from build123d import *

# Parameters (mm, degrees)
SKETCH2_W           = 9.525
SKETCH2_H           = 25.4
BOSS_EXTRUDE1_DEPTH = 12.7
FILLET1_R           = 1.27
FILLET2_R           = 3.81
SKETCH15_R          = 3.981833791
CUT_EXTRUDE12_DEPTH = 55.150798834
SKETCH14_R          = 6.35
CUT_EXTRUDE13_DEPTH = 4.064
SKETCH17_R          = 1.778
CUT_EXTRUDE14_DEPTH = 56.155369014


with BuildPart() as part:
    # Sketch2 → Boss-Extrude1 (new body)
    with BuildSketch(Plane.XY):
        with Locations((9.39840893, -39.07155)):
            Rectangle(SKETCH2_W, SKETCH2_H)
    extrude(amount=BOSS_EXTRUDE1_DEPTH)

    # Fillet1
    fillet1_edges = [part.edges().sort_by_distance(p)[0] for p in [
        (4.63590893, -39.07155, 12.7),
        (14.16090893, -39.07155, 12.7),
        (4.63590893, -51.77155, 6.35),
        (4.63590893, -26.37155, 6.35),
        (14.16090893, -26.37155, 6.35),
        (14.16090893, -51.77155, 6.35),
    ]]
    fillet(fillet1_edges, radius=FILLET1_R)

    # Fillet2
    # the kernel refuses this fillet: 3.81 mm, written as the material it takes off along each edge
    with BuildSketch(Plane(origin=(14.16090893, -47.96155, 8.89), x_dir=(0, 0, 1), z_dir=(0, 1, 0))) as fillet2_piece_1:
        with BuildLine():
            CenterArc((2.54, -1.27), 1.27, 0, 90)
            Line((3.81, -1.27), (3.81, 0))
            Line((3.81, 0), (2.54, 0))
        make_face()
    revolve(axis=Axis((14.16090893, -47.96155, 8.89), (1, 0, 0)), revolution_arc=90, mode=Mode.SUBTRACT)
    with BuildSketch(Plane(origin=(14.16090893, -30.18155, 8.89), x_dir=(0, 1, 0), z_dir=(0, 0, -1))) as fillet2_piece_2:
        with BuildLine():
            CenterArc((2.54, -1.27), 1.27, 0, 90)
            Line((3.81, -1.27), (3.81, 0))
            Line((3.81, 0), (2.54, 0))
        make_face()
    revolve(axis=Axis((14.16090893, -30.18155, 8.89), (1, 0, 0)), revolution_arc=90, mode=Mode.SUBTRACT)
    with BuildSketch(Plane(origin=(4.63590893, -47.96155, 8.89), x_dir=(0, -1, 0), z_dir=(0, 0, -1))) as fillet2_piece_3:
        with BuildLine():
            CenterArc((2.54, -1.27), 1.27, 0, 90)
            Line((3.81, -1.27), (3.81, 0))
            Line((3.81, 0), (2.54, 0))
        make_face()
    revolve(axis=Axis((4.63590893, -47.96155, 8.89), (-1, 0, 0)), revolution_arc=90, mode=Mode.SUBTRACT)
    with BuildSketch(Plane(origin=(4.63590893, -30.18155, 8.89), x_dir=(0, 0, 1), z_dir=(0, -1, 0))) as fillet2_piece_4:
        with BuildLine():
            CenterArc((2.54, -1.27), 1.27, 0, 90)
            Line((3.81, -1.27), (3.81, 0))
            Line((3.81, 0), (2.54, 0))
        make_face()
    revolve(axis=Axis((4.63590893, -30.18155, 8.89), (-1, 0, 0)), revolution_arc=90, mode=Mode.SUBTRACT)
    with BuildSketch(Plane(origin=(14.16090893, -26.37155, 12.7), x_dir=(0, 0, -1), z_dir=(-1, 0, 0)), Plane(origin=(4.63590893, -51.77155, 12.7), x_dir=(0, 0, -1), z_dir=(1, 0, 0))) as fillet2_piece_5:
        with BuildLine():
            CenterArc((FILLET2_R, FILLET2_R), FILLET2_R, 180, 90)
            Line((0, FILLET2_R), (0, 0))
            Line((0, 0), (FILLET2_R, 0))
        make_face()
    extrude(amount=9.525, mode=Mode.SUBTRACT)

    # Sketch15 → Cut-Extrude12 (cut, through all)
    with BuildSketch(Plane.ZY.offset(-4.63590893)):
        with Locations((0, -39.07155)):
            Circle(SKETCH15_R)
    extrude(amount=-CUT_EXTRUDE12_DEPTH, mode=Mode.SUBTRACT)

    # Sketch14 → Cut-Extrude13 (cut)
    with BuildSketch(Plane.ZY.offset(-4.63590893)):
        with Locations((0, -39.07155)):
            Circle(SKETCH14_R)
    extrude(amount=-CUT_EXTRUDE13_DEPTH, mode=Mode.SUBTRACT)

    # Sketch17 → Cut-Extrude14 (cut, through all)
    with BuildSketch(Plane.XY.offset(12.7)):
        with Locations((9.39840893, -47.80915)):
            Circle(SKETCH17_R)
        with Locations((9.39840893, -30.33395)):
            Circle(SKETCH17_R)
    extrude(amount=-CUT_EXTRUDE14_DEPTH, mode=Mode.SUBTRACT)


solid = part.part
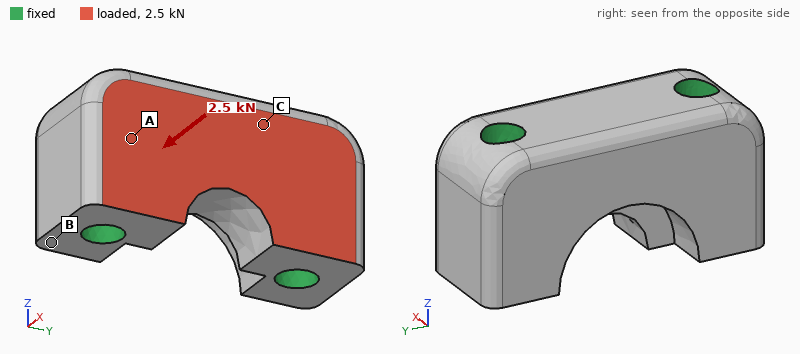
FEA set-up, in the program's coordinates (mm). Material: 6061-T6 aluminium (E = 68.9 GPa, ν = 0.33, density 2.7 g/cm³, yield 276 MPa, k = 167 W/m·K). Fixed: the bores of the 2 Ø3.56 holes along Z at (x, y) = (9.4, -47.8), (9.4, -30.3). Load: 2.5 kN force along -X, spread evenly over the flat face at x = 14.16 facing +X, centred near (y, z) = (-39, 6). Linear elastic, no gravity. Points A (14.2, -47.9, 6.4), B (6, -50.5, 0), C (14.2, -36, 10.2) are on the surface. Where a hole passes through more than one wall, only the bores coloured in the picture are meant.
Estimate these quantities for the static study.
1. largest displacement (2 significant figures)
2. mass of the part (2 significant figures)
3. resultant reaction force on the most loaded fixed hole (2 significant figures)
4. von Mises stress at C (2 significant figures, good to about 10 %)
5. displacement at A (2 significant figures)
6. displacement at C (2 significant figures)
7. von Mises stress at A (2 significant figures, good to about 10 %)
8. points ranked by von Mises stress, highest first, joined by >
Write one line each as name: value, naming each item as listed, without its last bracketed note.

largest displacement: 2.6 µm
mass of the part: 6.3 g
resultant reaction force on the most loaded fixed hole: 1.3 kN
von Mises stress at C: 7.5 MPa
displacement at A: 0.69 µm
displacement at C: 1.9 µm
von Mises stress at A: 14 MPa
points ranked by von Mises stress, highest first, joined by >: A > C > B
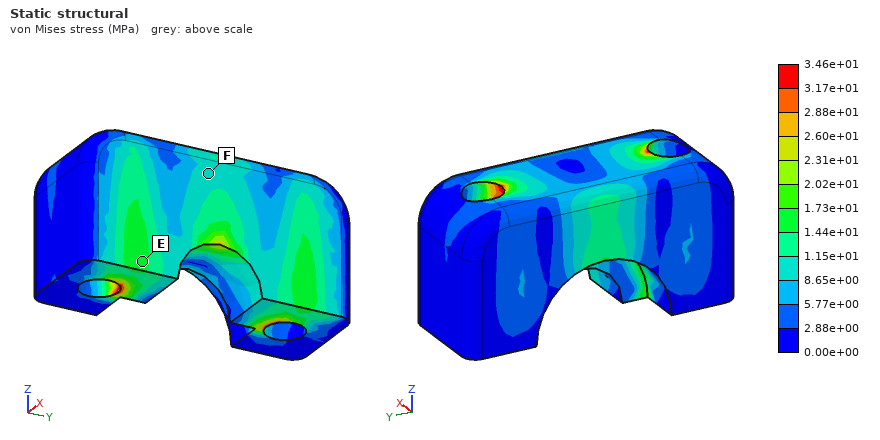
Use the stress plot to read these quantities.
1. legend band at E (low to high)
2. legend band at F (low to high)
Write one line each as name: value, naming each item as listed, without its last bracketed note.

legend band at E: 1.44e+01 to 1.73e+01 MPa
legend band at F: 8.65e+00 to 1.15e+01 MPa
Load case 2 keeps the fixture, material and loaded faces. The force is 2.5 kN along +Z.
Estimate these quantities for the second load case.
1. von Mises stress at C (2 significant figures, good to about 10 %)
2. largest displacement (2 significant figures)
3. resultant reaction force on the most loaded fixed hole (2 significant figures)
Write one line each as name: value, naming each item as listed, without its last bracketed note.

von Mises stress at C: 23 MPa
largest displacement: 4.9 µm
resultant reaction force on the most loaded fixed hole: 1.3 kN
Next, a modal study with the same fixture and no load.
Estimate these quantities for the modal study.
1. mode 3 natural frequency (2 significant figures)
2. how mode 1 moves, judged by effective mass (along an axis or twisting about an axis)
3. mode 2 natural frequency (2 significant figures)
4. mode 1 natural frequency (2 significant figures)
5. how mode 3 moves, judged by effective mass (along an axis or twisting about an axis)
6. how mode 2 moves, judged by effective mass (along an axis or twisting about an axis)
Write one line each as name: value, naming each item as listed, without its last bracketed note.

mode 3 natural frequency: 110 kHz
how mode 1 moves, judged by effective mass: along X
mode 2 natural frequency: 92 kHz
mode 1 natural frequency: 77 kHz
how mode 3 moves, judged by effective mass: twisting about Y
how mode 2 moves, judged by effective mass: along Z
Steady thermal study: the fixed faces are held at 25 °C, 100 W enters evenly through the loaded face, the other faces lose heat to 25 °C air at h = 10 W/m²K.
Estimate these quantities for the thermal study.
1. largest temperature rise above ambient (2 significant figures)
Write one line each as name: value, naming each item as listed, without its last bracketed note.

largest temperature rise above ambient: 16 K
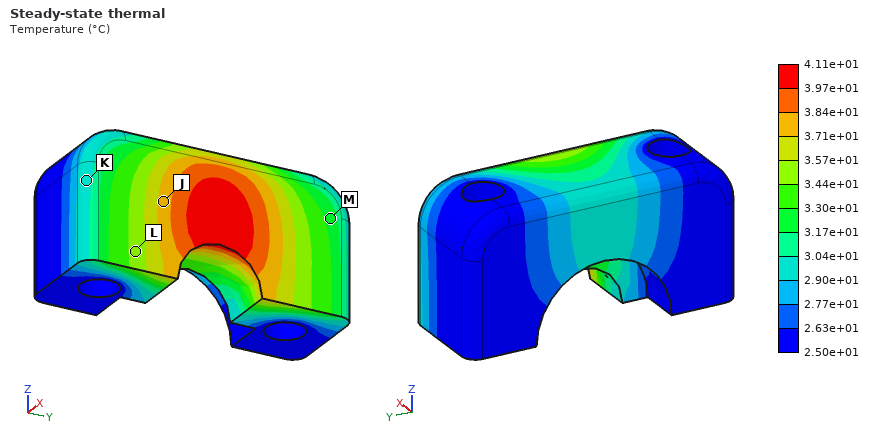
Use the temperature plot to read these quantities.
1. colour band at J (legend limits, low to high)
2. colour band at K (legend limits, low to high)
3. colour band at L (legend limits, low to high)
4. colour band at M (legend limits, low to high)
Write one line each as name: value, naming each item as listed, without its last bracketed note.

colour band at J: 3.71e+01 to 3.84e+01 °C
colour band at K: 2.90e+01 to 3.04e+01 °C
colour band at L: 3.44e+01 to 3.57e+01 °C
colour band at M: 3.17e+01 to 3.30e+01 °C
